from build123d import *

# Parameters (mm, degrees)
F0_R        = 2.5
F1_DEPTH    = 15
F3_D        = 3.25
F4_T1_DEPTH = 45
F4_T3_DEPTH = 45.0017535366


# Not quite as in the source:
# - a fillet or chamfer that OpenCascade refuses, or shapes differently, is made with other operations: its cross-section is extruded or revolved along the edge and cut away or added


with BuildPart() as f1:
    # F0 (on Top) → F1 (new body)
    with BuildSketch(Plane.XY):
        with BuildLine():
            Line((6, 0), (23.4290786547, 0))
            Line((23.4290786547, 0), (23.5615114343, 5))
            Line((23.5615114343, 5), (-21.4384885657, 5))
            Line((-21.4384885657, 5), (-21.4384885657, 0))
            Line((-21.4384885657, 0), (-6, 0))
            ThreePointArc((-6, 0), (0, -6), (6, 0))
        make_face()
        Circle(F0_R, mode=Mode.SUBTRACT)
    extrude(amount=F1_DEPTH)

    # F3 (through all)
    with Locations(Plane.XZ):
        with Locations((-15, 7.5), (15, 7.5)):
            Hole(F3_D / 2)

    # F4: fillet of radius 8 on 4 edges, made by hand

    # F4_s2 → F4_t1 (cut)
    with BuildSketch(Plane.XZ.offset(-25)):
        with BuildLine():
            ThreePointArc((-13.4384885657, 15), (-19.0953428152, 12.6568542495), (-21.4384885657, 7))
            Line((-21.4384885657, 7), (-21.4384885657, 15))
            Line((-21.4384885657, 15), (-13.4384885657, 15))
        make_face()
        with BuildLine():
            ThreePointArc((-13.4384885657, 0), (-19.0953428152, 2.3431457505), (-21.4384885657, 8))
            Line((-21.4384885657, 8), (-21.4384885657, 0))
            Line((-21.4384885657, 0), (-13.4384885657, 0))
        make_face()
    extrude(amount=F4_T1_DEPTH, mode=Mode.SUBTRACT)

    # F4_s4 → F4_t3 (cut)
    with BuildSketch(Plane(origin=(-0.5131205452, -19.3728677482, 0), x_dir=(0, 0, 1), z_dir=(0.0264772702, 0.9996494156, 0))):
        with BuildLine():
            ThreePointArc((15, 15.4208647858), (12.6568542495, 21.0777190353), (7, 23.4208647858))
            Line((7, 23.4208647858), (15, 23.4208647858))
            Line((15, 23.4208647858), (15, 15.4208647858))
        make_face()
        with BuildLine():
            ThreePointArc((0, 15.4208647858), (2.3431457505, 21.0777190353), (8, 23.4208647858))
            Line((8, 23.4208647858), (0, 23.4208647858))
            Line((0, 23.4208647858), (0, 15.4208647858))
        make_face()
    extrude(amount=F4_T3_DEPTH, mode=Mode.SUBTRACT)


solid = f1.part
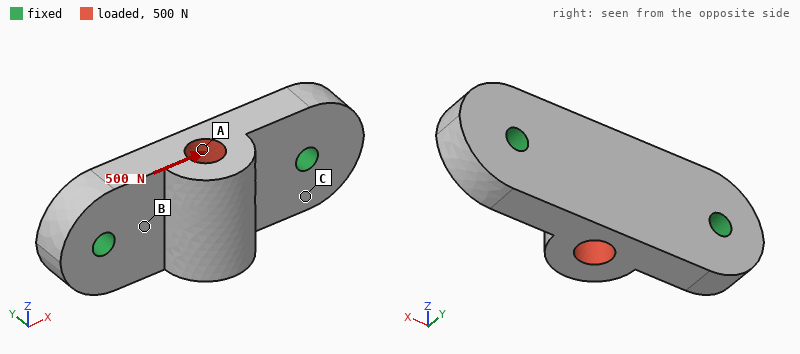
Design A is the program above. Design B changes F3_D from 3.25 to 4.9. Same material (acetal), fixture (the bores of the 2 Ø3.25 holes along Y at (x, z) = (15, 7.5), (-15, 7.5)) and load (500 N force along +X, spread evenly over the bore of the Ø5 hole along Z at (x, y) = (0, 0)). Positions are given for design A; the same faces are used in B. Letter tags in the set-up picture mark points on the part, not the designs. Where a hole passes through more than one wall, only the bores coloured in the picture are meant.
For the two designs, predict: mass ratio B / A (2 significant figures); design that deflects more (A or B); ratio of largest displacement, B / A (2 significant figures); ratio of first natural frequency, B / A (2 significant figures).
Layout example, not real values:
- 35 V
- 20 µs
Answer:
- 0.97
- A
- 0.88
- 1.1
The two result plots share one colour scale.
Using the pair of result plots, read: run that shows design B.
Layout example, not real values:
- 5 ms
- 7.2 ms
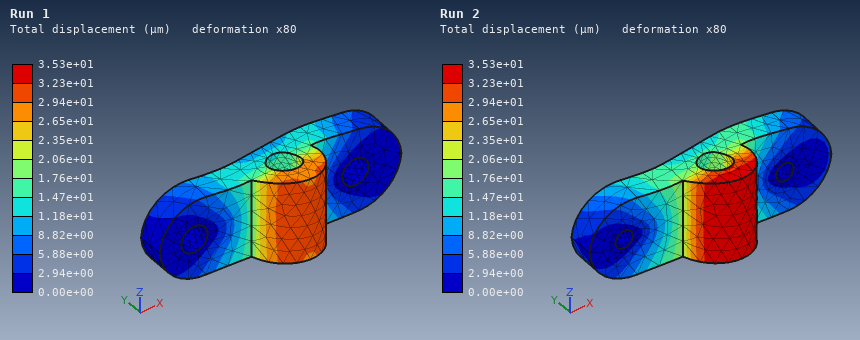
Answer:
- Run 1
